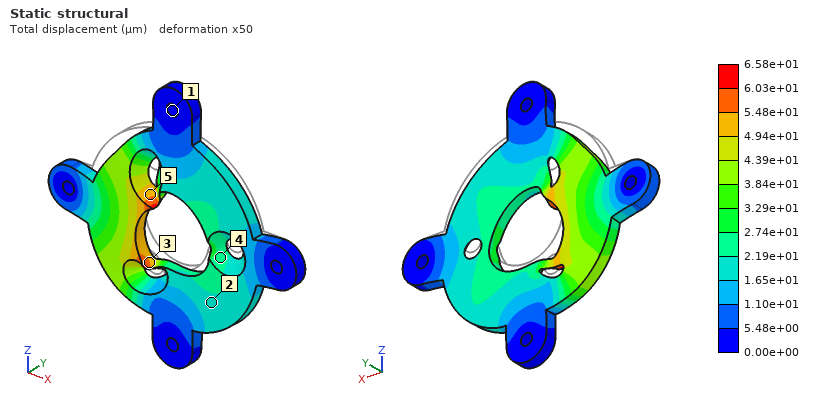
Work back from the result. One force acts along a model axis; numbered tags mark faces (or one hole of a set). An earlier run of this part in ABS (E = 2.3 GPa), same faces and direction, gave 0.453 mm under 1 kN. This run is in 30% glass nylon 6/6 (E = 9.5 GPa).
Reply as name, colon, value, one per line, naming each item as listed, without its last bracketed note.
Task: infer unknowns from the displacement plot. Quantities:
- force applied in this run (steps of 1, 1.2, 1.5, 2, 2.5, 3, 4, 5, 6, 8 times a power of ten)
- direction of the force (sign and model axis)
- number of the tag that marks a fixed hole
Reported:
force applied in this run: 600 N
direction of the force: -Z
number of the tag that marks a fixed hole: 1
